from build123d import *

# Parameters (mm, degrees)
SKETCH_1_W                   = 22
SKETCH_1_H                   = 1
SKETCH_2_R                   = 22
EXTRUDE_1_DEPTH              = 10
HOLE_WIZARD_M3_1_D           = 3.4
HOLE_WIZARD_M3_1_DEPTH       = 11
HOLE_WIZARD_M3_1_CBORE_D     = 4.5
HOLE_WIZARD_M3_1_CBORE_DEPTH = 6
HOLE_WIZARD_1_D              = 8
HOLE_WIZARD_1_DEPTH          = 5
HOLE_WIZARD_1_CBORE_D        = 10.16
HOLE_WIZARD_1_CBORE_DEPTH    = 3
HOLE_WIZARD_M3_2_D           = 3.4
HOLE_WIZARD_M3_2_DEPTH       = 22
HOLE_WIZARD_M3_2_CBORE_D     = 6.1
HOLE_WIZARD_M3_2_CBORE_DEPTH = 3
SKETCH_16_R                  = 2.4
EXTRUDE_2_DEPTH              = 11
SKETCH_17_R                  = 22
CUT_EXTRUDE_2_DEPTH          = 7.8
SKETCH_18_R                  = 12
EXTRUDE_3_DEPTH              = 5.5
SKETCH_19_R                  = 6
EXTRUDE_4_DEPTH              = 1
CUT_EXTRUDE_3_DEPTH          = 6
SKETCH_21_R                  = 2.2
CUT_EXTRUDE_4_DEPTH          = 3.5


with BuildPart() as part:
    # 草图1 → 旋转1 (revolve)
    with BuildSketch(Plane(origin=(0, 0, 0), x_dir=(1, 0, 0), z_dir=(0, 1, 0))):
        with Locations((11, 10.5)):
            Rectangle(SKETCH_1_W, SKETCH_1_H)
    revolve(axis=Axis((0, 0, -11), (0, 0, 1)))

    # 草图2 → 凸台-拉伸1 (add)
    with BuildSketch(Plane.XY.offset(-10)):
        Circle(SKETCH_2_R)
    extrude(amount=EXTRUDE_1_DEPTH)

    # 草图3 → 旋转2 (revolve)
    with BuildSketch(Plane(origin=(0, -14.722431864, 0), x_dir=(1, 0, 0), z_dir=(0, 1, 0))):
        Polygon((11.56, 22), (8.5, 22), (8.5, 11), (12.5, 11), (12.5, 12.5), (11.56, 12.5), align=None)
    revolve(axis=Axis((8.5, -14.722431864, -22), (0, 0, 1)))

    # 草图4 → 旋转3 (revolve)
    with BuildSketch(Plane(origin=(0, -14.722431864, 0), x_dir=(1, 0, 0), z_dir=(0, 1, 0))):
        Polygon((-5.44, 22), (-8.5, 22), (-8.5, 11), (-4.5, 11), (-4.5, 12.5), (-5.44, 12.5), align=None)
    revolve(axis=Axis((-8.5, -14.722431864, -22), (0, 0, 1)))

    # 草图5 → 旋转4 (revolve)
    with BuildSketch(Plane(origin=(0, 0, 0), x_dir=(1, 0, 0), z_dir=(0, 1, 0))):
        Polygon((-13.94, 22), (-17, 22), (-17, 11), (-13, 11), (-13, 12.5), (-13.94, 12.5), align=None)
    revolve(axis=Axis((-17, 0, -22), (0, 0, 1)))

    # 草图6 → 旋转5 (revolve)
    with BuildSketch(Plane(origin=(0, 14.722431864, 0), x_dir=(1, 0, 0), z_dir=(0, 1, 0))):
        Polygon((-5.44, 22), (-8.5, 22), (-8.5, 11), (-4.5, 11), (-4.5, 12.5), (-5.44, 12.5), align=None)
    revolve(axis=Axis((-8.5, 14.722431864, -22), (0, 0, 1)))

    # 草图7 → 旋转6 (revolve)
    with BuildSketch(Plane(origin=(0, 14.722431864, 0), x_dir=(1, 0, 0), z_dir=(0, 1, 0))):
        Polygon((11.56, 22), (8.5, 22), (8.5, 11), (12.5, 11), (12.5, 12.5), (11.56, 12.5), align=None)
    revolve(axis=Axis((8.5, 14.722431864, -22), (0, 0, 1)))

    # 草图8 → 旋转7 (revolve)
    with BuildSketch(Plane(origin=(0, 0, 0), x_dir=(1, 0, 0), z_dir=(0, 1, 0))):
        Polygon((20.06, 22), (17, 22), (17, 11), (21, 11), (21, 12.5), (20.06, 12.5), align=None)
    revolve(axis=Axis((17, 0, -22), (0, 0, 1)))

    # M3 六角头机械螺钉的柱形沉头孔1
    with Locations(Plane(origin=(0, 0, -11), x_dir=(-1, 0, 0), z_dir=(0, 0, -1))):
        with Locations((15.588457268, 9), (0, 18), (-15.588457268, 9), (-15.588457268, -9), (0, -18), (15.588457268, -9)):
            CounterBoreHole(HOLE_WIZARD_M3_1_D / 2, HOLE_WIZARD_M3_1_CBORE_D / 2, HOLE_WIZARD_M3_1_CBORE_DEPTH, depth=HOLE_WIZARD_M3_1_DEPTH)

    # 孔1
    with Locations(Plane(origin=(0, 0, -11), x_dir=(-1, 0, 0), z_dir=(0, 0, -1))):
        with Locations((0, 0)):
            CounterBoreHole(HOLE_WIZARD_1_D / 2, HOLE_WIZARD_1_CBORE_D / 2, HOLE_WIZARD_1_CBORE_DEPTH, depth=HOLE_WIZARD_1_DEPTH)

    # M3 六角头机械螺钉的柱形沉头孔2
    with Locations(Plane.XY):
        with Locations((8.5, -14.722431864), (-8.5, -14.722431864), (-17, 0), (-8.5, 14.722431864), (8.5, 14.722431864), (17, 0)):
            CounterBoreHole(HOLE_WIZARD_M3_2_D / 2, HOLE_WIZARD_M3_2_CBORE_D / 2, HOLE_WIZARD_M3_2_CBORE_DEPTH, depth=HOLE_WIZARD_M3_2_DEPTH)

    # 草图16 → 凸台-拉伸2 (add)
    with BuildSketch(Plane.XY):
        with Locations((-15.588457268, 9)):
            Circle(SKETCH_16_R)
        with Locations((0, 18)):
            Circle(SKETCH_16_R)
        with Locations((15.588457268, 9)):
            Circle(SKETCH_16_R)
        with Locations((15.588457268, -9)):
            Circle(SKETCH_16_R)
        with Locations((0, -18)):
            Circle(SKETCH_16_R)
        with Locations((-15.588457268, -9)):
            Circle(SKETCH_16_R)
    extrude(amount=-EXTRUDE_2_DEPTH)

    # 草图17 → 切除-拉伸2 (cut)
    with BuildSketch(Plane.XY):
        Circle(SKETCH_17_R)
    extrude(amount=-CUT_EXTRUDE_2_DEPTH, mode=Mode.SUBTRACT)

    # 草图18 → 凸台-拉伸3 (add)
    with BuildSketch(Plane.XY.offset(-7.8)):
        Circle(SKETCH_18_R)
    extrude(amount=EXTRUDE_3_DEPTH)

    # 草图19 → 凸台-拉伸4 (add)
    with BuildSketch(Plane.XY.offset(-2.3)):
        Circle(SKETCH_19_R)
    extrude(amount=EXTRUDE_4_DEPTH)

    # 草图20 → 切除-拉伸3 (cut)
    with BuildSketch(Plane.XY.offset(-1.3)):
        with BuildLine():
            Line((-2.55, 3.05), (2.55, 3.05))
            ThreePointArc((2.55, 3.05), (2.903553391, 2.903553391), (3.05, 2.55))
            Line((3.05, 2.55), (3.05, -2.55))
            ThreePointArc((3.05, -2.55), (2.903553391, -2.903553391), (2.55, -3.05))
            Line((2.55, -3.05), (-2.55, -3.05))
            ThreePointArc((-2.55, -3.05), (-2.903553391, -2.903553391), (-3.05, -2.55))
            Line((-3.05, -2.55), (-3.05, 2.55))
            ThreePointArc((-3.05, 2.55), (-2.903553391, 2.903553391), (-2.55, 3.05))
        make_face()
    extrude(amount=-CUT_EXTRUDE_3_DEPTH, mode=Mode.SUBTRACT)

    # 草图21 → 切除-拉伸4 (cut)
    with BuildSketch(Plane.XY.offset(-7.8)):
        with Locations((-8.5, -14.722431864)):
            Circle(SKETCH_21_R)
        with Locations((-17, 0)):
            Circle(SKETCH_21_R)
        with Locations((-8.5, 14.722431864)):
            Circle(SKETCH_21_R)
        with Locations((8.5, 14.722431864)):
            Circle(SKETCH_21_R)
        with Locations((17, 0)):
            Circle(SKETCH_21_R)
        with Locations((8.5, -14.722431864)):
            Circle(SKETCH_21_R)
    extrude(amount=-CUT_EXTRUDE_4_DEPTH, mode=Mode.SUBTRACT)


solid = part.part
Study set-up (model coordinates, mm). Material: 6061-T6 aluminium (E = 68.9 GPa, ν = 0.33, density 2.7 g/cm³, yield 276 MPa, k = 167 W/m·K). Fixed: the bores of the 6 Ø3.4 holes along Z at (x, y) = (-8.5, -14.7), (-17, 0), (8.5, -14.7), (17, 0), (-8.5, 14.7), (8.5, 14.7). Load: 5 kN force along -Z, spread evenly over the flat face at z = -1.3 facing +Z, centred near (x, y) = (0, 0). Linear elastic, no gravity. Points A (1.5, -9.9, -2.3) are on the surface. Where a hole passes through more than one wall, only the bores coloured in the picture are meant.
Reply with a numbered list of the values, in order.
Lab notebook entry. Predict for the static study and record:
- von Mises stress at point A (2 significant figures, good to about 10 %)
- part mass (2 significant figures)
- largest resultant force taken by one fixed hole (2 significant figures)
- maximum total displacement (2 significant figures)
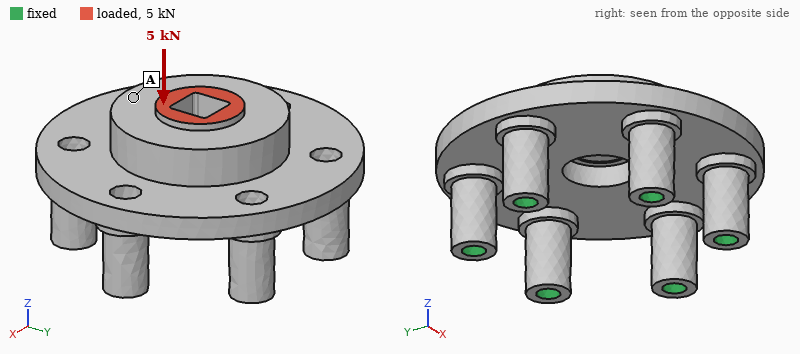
1. 23 MPa
2. 22 g
3. 1.2 kN
4. 23 µm
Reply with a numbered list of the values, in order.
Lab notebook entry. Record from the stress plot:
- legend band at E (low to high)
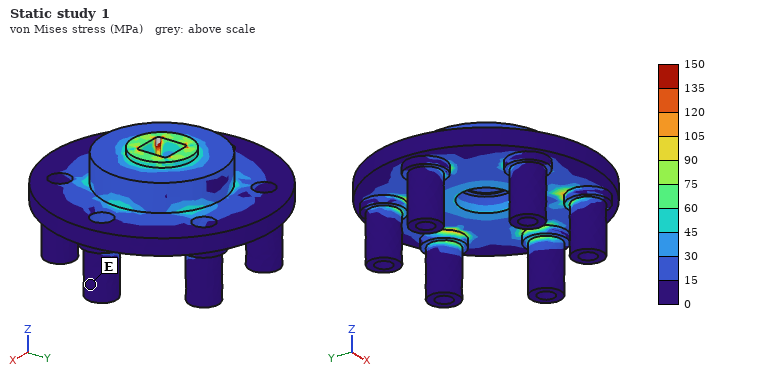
1. 0 to 15 MPa
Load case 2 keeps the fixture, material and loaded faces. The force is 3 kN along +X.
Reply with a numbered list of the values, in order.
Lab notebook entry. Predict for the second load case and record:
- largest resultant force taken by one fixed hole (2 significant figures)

1. 1.0 kN
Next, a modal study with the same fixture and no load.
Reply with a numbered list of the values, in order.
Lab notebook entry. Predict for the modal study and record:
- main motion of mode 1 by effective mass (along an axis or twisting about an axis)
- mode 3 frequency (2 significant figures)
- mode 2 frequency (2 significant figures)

1. along Z
2. 33 kHz
3. 33 kHz
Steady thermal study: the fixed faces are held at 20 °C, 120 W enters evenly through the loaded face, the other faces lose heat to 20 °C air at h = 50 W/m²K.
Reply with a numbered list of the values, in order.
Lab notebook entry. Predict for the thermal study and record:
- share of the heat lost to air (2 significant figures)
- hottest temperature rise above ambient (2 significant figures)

1. 3.3 %
2. 64 K
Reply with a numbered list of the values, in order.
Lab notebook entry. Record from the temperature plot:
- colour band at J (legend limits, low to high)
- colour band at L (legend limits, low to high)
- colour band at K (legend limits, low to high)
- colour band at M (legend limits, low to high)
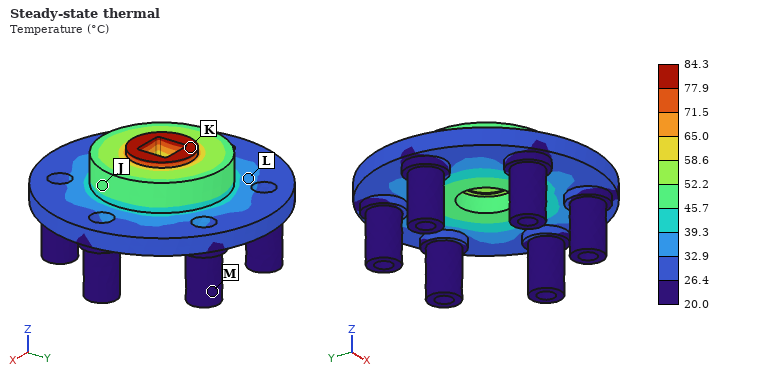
1. 45.7 to 52.2 °C
2. 32.9 to 39.3 °C
3. 77.9 to 84.3 °C
4. 20.0 to 26.4 °C
